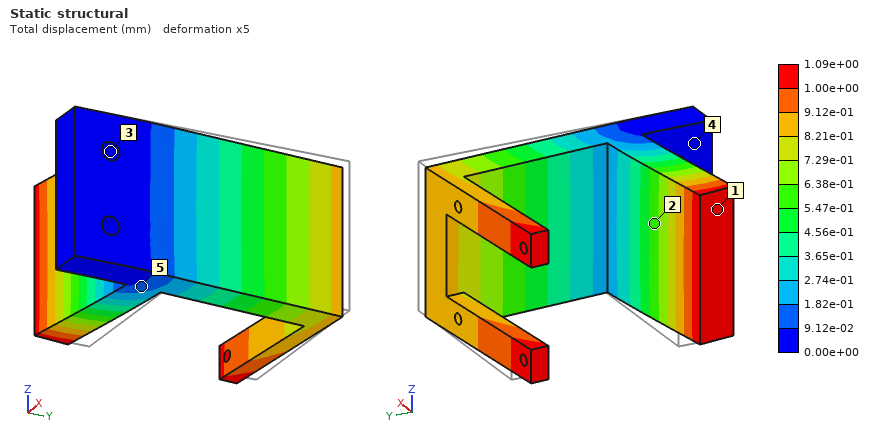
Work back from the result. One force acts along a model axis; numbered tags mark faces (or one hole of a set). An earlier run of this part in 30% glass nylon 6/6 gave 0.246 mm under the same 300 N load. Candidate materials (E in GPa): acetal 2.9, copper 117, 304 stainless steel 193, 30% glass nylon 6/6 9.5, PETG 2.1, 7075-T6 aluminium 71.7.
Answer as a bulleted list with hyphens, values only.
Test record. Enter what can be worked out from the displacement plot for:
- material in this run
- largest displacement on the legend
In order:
- PETG
- 1.09e+00 mm
